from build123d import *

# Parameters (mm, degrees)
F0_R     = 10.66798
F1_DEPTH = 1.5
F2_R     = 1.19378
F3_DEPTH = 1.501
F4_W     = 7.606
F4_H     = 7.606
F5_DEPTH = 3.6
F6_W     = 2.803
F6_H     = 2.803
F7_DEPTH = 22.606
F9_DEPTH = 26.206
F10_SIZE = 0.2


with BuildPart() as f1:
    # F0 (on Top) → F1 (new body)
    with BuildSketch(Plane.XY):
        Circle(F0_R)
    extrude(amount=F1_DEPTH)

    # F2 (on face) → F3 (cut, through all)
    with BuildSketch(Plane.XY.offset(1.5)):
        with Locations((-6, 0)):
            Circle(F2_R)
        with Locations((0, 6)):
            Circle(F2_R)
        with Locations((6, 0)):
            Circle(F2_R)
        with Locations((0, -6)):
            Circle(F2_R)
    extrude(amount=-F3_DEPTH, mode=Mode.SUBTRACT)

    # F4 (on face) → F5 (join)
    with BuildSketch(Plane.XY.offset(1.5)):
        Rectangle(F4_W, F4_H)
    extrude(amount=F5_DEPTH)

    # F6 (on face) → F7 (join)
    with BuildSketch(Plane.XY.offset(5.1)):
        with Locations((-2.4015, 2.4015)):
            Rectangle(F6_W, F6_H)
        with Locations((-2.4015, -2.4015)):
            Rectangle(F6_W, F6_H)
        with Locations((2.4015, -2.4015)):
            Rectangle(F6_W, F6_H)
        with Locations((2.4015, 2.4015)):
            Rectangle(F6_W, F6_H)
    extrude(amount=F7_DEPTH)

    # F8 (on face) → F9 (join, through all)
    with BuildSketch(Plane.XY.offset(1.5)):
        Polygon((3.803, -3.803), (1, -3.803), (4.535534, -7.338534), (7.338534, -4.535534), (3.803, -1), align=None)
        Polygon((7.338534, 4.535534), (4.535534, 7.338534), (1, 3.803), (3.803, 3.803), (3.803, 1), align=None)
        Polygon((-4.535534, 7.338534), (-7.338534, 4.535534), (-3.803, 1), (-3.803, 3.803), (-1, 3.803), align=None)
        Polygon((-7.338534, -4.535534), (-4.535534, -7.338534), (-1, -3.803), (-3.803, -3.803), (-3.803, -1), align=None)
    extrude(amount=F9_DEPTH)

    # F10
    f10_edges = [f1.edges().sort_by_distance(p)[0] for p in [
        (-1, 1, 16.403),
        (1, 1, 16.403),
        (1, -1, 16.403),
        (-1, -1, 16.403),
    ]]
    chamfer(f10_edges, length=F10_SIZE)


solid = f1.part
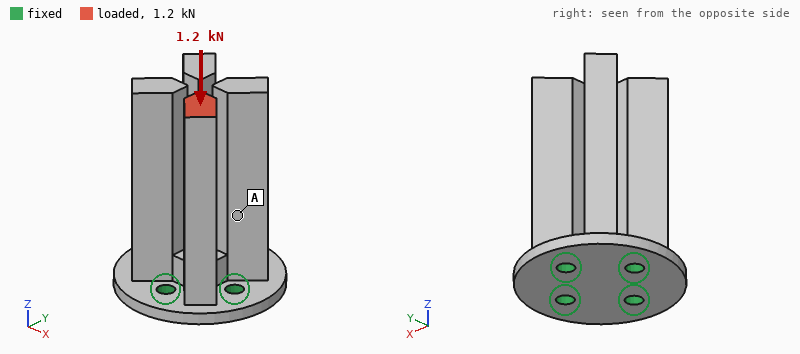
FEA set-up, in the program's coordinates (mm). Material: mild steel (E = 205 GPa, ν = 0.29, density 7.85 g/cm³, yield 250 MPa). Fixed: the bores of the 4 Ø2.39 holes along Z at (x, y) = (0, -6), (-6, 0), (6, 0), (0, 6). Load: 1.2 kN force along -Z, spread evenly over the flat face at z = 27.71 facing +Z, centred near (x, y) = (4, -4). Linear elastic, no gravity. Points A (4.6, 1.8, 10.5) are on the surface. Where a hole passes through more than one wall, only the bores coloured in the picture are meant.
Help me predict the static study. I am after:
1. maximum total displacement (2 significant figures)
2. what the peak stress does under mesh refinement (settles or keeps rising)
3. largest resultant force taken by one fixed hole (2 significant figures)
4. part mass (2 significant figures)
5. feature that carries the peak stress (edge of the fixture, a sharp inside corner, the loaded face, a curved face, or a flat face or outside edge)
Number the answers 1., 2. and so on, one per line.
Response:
1. 23 µm
2. keeps rising
3. 680 N
4. 24 g
5. edge of the fixture
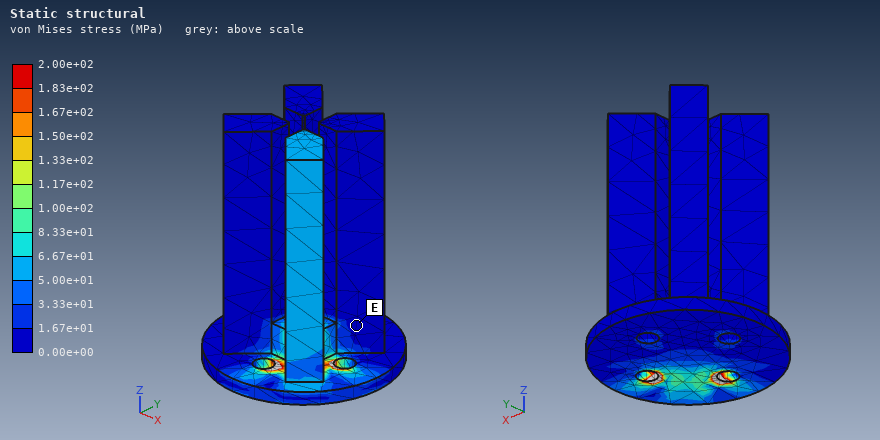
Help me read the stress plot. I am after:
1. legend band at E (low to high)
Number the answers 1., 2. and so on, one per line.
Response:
1. 0.00e+00 to 1.67e+01 MPa
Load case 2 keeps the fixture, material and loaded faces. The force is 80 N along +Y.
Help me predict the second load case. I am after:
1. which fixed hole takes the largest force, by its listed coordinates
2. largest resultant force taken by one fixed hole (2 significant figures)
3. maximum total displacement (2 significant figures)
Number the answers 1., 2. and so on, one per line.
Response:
1. (0, -6)
2. 230 N
3. 64 µm
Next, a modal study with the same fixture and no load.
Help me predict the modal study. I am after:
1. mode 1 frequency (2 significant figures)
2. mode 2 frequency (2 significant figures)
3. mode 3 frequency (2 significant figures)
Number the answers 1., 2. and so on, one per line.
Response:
1. 4500 Hz
2. 4500 Hz
3. 4600 Hz
